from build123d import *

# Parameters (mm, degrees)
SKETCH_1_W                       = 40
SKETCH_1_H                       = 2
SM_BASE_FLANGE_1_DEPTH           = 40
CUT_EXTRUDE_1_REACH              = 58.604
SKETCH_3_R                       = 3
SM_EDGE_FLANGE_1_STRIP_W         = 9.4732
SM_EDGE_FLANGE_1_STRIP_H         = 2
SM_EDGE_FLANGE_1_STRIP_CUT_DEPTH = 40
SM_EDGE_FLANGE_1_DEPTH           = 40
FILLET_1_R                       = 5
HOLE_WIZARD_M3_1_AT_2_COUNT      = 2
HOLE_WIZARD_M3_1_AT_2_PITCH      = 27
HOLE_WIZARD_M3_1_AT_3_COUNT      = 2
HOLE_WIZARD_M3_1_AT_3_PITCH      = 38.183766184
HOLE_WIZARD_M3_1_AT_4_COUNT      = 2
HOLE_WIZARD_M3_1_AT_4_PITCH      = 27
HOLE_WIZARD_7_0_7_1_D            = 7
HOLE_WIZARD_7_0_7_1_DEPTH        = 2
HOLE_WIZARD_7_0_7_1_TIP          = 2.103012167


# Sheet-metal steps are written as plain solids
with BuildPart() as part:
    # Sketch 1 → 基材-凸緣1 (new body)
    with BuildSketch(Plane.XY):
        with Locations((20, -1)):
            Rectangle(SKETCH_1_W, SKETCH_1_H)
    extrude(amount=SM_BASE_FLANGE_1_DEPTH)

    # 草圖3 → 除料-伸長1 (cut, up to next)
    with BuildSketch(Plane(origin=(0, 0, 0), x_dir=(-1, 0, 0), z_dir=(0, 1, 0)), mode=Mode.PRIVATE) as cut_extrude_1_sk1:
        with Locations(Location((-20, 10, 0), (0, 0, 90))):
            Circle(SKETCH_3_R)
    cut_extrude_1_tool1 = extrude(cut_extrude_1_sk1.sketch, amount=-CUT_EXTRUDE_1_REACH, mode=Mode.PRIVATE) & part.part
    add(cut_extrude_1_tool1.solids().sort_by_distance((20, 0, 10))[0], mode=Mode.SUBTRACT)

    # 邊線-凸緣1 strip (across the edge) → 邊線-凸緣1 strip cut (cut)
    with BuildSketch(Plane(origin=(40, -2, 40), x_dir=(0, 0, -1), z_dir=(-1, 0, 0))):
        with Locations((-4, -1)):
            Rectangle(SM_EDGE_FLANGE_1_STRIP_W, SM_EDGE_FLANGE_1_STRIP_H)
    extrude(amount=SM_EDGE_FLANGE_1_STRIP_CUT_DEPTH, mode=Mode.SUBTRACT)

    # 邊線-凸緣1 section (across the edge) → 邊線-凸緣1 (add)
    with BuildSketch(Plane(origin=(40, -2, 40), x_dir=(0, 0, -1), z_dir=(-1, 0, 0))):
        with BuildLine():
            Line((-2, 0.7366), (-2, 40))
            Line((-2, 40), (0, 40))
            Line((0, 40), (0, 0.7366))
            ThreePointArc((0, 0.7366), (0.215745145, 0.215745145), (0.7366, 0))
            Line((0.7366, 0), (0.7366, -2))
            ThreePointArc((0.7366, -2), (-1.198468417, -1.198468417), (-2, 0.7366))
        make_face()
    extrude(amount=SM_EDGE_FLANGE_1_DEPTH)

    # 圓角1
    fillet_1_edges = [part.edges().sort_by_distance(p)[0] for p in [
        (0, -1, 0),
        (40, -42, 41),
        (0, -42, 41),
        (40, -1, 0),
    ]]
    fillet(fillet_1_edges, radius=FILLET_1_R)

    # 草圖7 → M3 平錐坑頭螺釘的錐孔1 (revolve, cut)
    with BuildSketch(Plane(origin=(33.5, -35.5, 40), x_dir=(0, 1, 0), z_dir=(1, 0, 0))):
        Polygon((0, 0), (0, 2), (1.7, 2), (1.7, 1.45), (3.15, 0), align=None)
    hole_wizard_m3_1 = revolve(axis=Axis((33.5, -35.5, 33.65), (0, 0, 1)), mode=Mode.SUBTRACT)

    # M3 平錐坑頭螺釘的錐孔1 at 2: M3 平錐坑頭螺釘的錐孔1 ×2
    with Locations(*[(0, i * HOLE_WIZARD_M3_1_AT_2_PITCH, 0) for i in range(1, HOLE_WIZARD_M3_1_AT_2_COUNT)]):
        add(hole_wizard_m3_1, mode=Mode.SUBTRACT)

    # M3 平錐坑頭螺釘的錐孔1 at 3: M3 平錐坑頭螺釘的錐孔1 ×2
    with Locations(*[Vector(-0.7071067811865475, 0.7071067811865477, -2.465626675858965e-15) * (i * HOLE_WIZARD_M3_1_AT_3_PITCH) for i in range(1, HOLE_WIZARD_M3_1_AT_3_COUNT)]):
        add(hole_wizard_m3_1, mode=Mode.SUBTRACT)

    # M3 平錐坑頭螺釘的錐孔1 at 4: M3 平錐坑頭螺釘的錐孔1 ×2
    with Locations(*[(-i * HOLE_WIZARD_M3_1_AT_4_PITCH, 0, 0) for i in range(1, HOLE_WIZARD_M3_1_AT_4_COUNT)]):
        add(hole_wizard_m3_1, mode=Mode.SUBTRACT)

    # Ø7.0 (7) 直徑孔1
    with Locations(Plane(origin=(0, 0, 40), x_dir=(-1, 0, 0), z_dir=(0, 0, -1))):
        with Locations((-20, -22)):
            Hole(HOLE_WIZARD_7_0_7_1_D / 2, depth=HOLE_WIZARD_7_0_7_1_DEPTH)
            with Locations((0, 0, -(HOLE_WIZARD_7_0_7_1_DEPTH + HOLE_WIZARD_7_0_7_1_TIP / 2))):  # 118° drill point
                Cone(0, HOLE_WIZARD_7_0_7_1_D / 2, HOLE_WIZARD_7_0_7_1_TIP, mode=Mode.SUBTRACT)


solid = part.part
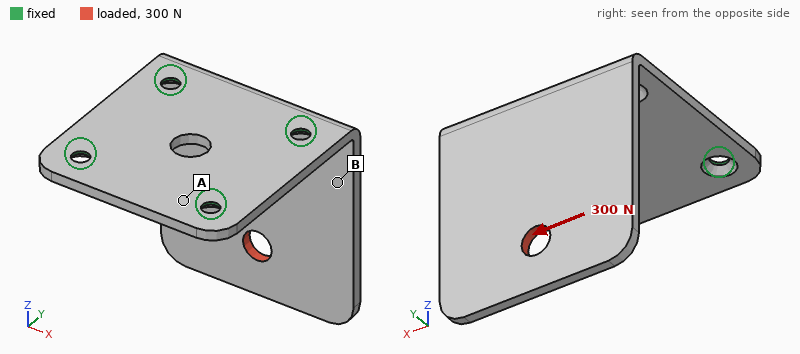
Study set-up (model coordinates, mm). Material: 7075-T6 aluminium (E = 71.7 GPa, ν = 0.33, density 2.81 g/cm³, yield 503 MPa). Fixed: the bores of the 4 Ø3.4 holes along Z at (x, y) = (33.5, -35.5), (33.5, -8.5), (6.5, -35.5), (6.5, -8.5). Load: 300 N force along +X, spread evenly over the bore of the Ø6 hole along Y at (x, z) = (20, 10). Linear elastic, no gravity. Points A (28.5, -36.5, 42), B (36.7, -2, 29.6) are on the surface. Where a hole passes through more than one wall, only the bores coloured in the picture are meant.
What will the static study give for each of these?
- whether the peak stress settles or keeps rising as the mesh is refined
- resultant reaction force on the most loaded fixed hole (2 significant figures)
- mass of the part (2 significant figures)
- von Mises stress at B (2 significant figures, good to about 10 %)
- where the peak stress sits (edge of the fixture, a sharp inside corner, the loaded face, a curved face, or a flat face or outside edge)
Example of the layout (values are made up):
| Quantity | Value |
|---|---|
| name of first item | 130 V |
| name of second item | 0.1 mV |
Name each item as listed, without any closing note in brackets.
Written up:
| Quantity | Value |
|---|---|
| whether the peak stress settles or keeps rising as the mesh is refined | keeps rising |
| resultant reaction force on the most loaded fixed hole | 470 N |
| mass of the part | 17 g |
| von Mises stress at B | 42 MPa |
| where the peak stress sits | edge of the fixture |
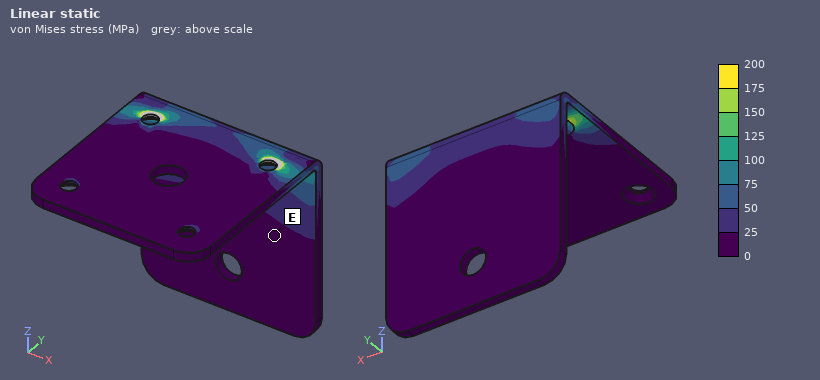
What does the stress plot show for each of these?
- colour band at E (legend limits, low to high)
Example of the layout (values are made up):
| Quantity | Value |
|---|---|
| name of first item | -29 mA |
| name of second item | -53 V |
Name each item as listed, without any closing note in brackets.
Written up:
| Quantity | Value |
|---|---|
| colour band at E | 0 to 25 MPa |
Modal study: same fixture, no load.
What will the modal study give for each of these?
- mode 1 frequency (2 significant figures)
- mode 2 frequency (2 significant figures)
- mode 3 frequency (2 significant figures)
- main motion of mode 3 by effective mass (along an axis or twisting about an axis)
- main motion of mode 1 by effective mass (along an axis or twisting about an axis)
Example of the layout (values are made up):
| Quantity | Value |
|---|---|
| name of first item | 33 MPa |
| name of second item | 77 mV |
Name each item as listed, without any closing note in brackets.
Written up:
| Quantity | Value |
|---|---|
| mode 1 frequency | 720 Hz |
| mode 2 frequency | 2000 Hz |
| mode 3 frequency | 3200 Hz |
| main motion of mode 3 by effective mass | along X |
| main motion of mode 1 by effective mass | along Y |
